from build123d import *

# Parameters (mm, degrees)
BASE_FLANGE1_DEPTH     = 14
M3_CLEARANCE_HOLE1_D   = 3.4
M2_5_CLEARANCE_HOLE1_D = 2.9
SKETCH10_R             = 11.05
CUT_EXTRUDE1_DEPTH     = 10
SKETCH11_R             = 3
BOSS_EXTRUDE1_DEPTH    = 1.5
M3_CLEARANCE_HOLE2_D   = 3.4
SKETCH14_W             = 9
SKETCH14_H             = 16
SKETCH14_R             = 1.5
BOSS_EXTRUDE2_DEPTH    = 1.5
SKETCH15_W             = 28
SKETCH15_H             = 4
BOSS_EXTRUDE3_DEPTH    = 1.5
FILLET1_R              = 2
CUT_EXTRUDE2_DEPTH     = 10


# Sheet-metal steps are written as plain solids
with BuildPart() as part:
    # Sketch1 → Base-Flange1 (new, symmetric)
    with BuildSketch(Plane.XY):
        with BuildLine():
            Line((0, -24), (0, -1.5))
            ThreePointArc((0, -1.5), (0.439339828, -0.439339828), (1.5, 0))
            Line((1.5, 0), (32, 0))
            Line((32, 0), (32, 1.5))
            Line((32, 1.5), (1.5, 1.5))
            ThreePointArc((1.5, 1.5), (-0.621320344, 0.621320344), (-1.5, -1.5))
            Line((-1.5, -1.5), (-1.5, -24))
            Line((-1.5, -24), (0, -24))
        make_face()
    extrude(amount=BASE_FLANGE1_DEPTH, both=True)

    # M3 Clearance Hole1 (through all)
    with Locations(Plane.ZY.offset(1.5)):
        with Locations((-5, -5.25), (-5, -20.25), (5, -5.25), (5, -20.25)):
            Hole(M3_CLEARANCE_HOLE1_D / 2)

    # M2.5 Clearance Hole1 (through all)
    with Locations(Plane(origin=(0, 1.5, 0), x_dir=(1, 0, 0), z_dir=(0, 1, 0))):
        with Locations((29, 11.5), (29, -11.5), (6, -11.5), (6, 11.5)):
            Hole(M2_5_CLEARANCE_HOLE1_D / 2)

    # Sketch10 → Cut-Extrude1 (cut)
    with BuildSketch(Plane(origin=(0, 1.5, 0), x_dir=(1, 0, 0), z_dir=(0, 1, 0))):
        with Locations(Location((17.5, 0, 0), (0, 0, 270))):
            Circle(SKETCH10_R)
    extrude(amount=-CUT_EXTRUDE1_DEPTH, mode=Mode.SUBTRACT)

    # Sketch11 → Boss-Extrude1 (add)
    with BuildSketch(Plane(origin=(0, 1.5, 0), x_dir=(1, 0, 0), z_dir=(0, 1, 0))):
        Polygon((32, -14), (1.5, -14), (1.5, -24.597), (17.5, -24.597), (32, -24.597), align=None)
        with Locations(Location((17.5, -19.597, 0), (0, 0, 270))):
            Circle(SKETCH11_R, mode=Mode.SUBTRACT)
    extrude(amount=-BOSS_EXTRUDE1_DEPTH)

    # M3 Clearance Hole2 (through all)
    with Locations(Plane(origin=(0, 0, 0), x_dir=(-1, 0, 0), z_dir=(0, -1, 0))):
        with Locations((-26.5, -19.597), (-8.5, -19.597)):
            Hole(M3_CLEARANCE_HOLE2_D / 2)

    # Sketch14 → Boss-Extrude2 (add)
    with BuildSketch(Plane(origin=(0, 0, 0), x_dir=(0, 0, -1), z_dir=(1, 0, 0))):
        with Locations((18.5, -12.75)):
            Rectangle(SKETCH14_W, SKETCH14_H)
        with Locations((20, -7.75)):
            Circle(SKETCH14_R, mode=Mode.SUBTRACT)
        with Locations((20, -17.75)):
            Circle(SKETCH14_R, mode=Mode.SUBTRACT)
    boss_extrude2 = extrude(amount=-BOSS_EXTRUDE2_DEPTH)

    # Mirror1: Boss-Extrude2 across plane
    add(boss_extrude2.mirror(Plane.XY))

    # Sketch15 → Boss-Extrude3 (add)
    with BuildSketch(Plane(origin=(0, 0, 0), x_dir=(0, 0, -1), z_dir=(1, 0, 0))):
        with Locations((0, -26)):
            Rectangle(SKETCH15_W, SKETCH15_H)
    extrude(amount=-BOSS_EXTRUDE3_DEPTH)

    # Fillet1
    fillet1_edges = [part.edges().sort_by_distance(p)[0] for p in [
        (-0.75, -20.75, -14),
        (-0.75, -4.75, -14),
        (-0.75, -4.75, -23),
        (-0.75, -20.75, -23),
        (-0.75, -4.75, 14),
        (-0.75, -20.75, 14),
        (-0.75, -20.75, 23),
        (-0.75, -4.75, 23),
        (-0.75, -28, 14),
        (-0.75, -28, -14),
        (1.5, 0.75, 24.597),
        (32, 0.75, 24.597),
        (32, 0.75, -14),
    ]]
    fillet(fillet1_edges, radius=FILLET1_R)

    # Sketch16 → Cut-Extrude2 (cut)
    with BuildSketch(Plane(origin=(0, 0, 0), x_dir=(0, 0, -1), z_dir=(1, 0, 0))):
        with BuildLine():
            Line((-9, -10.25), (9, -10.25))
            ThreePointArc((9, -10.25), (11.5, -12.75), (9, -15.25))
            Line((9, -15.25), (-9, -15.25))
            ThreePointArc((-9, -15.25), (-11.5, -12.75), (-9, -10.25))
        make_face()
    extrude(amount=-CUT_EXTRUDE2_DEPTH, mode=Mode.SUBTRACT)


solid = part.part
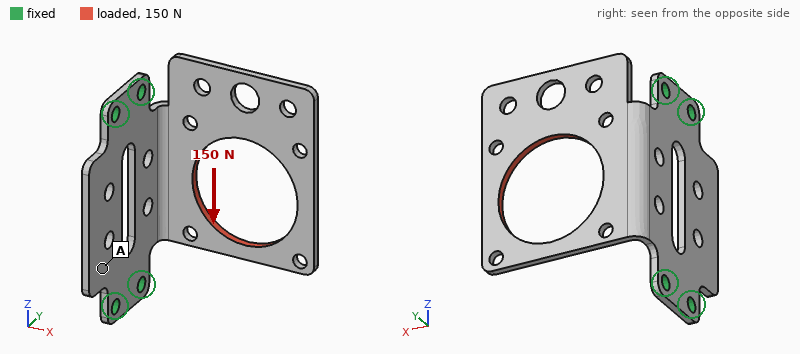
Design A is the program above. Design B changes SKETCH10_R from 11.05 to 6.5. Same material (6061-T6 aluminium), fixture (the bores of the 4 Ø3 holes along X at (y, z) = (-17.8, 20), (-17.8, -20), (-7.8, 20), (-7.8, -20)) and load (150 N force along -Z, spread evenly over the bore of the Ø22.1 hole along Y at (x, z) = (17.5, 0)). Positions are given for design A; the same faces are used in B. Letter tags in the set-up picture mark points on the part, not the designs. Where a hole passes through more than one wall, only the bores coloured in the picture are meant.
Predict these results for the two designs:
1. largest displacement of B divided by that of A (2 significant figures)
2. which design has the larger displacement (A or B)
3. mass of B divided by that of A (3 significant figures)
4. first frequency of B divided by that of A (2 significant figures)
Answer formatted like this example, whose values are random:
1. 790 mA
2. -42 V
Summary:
1. 0.89
2. A
3. 1.15
4. 0.97
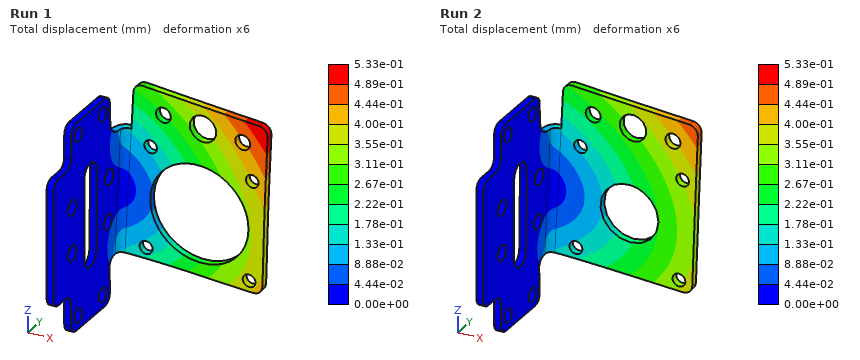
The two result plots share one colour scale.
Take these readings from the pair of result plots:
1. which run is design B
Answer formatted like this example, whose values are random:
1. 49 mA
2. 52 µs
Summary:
1. Run 2
